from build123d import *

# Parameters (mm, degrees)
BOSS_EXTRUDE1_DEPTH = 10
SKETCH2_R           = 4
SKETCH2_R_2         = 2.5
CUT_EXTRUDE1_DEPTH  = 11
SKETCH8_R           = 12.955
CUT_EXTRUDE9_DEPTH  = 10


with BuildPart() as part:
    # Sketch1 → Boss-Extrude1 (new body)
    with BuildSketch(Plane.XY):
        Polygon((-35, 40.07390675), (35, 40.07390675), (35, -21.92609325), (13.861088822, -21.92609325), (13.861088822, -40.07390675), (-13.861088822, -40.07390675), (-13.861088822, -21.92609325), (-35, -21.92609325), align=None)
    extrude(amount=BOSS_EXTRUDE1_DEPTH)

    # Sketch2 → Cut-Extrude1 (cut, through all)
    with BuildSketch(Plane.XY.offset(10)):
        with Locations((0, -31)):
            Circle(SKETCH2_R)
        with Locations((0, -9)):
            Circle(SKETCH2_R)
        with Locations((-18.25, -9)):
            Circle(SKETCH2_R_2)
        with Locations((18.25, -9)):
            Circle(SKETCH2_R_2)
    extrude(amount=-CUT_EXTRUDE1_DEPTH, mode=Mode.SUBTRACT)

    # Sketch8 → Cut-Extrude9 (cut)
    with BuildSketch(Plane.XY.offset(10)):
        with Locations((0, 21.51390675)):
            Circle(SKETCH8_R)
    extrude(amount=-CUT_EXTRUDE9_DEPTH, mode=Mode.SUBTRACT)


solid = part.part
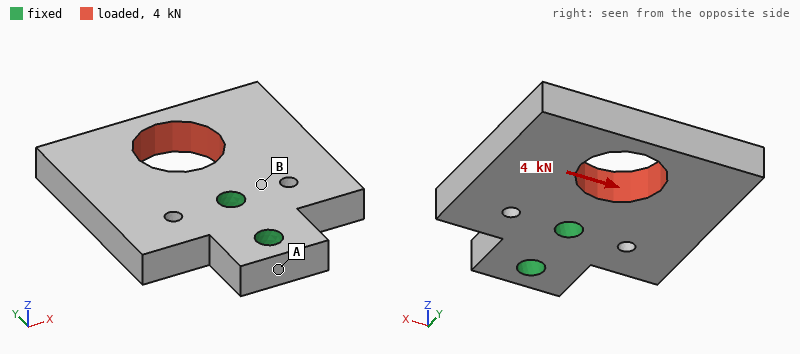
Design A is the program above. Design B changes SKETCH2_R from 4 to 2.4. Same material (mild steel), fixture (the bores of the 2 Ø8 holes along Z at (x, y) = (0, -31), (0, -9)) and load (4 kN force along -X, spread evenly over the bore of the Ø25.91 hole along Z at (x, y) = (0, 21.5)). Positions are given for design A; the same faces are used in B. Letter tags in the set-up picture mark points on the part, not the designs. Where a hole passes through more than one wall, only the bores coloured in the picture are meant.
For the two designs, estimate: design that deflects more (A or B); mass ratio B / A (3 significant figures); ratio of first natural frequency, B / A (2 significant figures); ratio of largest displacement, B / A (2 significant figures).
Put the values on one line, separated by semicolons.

B; 1.02; 0.92; 1.2
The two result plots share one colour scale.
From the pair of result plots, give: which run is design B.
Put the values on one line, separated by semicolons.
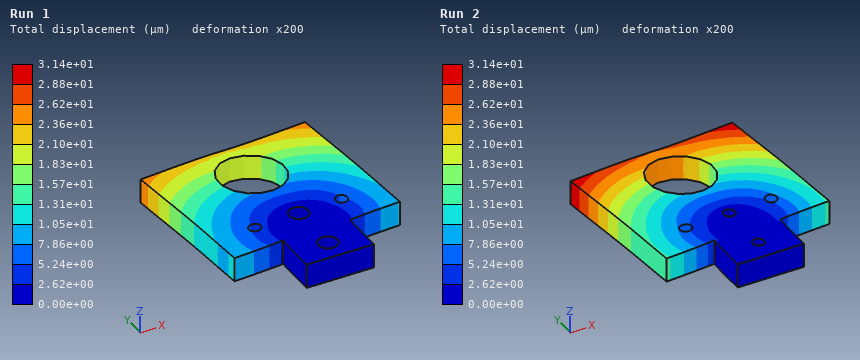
Run 2
